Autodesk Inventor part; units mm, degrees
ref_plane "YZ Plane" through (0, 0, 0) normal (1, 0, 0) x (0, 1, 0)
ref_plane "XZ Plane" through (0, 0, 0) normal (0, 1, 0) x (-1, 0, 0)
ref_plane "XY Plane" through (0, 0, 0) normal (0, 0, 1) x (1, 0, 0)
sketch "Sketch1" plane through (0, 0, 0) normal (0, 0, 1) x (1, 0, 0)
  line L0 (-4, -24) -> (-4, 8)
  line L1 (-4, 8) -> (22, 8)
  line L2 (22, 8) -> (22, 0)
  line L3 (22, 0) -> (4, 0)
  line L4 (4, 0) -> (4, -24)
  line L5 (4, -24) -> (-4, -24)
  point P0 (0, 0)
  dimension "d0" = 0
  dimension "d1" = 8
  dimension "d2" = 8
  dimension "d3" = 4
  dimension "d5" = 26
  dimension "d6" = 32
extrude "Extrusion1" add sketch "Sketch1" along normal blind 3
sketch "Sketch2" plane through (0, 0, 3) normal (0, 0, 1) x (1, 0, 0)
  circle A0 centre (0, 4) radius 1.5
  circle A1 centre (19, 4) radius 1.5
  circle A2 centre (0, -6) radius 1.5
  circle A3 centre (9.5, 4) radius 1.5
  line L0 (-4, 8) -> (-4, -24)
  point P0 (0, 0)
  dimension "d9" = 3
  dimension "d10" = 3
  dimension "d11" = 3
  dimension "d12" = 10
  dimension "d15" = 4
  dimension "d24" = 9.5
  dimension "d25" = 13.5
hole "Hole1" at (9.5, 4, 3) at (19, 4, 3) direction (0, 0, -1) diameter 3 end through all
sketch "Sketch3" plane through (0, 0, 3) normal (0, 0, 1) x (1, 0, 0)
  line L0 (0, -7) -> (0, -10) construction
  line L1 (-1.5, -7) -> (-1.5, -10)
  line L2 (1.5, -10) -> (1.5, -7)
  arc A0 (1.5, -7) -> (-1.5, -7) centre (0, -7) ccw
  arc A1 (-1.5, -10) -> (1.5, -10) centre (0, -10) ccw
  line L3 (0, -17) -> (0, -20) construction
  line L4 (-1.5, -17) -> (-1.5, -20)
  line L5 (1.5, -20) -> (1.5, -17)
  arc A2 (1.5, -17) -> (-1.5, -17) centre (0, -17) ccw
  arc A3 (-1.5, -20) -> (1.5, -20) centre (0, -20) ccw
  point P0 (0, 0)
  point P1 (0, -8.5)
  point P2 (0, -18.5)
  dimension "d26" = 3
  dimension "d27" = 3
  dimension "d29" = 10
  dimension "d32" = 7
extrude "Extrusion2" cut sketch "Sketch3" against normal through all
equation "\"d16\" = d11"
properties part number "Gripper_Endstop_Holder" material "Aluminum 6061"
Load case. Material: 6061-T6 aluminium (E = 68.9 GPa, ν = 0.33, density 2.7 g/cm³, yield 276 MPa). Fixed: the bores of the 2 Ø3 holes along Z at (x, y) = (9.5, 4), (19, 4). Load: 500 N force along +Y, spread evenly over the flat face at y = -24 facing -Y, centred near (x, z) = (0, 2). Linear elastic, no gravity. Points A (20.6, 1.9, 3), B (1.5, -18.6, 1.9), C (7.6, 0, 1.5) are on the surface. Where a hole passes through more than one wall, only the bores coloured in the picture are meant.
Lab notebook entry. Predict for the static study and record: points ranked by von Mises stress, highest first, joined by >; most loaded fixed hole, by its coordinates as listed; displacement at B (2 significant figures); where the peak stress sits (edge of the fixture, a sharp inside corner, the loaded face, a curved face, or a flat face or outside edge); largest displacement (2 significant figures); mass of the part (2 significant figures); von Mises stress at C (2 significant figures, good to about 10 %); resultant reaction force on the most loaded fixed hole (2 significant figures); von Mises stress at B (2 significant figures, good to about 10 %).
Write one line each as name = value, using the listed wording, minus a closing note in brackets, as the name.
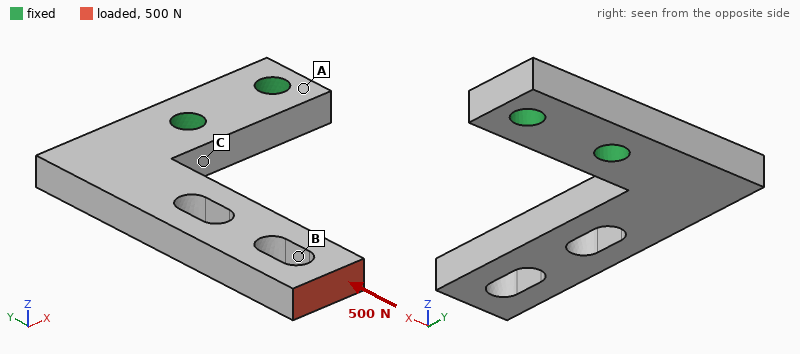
points ranked by von Mises stress, highest first, joined by > = C > B > A
most loaded fixed hole, by its coordinates as listed = (9.5, 4)
displacement at B = 0.091 mm
where the peak stress sits = edge of the fixture
largest displacement = 0.12 mm
mass of the part = 2.9 g
von Mises stress at C = 120 MPa
resultant reaction force on the most loaded fixed hole = 680 N
von Mises stress at B = 49 MPa
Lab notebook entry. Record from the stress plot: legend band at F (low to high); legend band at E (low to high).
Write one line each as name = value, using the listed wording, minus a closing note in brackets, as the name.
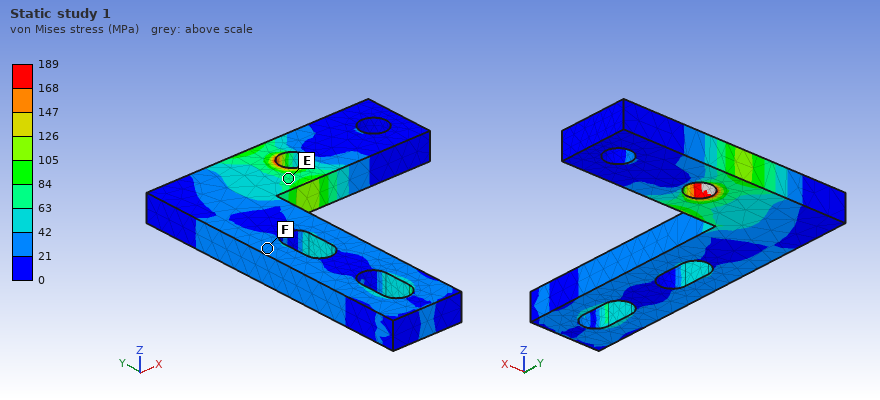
legend band at F = 21 to 42 MPa
legend band at E = 63 to 84 MPa
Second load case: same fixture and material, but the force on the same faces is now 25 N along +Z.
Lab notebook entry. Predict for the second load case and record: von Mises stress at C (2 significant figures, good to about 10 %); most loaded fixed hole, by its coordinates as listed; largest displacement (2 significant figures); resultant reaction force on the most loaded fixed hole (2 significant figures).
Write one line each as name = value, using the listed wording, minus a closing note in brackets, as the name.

von Mises stress at C = 41 MPa
most loaded fixed hole, by its coordinates as listed = (9.5, 4)
largest displacement = 0.24 mm
resultant reaction force on the most loaded fixed hole = 28 N
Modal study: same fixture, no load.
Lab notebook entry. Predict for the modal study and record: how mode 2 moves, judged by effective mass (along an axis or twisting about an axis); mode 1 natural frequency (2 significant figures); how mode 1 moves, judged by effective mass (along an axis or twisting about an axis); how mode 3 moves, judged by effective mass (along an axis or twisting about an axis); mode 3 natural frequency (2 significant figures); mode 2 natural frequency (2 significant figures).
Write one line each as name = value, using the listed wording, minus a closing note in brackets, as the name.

how mode 2 moves, judged by effective mass = along X
mode 1 natural frequency = 2600 Hz
how mode 1 moves, judged by effective mass = along Z
how mode 3 moves, judged by effective mass = along Z
mode 3 natural frequency = 9500 Hz
mode 2 natural frequency = 5600 Hz
